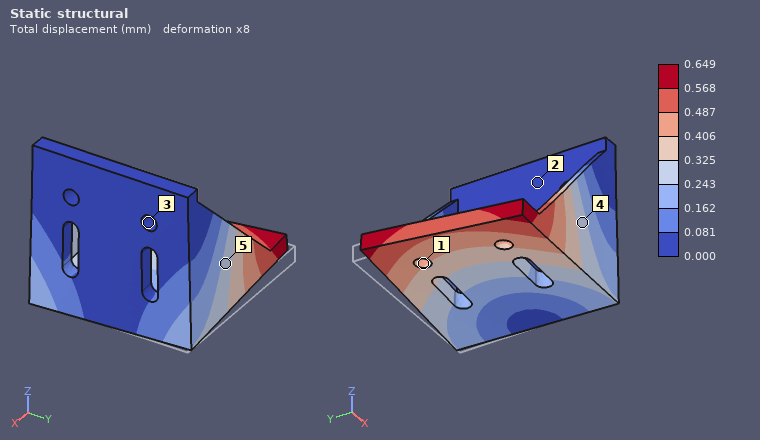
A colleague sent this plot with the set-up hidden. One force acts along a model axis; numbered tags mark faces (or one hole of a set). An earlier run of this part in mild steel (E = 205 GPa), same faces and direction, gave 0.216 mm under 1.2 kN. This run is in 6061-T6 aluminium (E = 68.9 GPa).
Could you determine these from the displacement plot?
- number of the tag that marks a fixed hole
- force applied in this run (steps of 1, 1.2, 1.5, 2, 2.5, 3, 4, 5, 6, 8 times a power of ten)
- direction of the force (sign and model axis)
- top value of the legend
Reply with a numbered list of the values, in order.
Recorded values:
1. 3
2. 1.2 kN
3. -Y
4. 0.649 mm
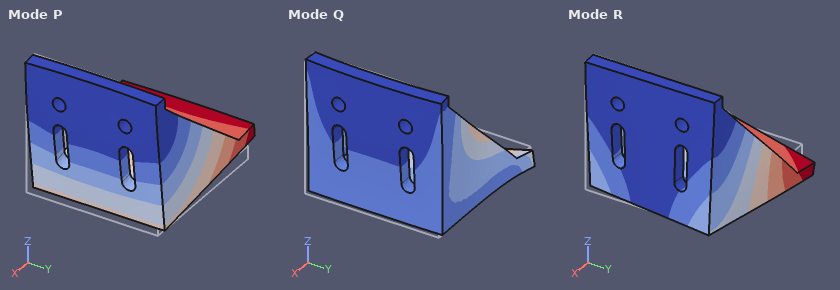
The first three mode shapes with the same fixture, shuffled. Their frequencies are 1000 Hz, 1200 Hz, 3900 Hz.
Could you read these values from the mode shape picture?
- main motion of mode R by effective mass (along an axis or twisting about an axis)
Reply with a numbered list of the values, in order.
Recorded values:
1. along Y
